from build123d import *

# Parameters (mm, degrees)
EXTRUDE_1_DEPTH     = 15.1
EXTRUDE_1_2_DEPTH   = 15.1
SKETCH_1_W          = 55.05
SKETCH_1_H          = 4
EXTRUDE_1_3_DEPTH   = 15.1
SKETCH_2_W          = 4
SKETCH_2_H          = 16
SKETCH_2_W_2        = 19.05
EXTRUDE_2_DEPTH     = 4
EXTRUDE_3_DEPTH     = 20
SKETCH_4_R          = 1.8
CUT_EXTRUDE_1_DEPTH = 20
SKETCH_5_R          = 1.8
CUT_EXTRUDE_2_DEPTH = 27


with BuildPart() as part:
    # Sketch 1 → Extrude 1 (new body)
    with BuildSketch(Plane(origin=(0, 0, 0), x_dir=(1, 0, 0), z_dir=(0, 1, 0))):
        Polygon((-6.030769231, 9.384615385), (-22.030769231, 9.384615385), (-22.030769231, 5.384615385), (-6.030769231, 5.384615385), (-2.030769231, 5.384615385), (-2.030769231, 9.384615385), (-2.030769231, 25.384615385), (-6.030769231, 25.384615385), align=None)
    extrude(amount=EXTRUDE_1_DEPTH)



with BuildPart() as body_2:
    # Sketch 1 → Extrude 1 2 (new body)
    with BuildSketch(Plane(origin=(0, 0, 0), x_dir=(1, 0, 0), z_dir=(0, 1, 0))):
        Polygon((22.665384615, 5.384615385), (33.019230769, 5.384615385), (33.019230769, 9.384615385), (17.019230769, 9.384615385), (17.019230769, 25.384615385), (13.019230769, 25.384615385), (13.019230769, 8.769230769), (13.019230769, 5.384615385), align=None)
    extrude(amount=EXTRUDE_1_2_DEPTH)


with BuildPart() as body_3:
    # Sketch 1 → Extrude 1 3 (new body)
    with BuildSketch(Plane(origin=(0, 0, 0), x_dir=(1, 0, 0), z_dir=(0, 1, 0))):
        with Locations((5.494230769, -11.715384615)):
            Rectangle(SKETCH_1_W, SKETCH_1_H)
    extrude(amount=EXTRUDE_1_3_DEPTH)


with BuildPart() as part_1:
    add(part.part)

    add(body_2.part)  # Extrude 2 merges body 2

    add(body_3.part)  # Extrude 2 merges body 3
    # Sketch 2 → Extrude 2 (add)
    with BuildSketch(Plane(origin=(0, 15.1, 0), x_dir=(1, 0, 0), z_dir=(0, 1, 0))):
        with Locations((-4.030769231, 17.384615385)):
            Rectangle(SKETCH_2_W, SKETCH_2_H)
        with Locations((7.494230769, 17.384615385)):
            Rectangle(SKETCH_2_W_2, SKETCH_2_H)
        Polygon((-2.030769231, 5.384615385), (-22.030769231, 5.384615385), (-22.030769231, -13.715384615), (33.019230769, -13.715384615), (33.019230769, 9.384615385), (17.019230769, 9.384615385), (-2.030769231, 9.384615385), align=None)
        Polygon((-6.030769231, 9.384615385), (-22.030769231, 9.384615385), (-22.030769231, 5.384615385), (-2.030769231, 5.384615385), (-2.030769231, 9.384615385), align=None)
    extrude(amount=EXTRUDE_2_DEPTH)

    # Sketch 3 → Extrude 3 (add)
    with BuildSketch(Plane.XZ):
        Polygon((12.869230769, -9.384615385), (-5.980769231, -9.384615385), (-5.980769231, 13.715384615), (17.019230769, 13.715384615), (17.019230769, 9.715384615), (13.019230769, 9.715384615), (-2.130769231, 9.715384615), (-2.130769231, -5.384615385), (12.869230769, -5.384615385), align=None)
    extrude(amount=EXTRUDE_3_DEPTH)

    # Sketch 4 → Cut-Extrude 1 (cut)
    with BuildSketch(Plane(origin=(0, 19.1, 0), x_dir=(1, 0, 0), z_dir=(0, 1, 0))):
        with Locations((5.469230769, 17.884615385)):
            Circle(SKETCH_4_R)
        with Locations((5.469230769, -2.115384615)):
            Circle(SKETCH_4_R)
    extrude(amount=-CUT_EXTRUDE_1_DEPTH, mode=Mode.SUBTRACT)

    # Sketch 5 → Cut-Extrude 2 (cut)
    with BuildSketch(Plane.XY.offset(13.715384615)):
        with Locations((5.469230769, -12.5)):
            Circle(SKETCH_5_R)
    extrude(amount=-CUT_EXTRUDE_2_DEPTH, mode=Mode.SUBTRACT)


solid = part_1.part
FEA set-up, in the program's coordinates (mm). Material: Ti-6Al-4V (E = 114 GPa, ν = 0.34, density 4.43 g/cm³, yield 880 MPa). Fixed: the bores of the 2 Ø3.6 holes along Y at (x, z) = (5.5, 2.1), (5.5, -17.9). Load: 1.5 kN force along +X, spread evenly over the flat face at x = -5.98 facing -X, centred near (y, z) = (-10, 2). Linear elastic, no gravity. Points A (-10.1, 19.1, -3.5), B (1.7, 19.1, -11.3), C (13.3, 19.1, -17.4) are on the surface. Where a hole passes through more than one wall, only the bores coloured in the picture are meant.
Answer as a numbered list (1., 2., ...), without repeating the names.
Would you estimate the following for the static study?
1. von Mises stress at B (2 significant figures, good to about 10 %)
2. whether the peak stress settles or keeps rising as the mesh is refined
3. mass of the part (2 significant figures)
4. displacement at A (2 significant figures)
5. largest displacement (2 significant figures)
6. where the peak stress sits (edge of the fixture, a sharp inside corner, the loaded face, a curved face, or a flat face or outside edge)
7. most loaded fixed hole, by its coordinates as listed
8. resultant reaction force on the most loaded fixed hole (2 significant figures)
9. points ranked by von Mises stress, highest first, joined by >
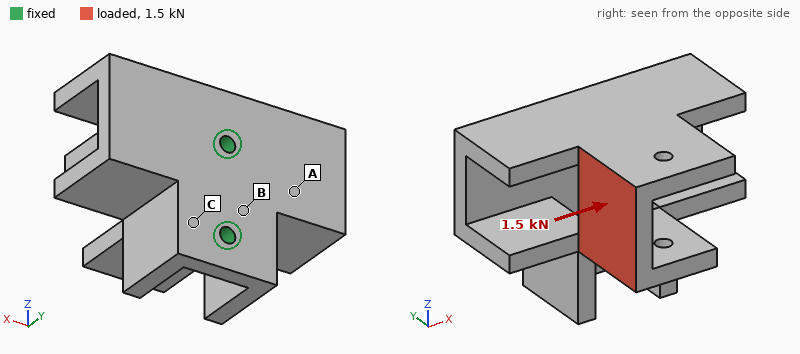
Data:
1. 130 MPa
2. keeps rising
3. 82 g
4. 0.11 mm
5. 0.49 mm
6. edge of the fixture
7. (5.5, 2.1)
8. 1.4 kN
9. B > C > A
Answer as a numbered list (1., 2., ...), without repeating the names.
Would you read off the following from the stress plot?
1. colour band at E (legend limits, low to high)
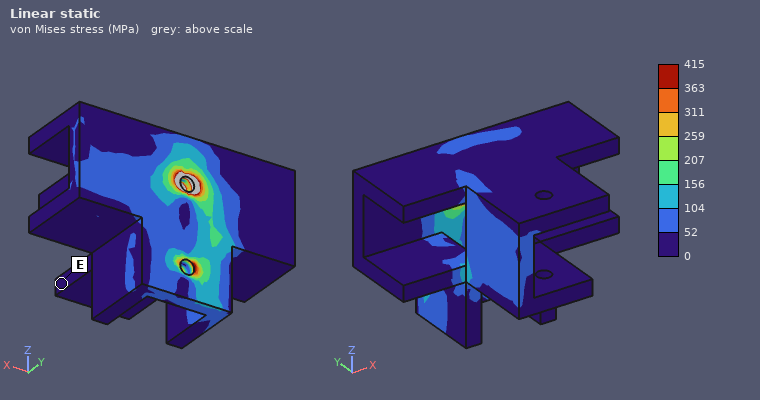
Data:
1. 0 to 52 MPa
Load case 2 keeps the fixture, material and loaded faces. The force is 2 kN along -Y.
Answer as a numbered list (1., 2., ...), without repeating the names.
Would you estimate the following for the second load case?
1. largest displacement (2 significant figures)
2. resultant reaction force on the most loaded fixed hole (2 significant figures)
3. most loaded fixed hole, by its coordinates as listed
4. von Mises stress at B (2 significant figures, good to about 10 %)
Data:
1. 0.20 mm
2. 1.7 kN
3. (5.5, 2.1)
4. 66 MPa
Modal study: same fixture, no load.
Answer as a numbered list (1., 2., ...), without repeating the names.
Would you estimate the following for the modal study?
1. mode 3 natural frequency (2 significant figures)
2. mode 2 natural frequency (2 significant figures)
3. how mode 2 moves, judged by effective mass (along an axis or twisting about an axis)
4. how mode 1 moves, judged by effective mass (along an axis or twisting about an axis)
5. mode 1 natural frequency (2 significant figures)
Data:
1. 5000 Hz
2. 3300 Hz
3. along Z
4. along X
5. 1900 Hz
